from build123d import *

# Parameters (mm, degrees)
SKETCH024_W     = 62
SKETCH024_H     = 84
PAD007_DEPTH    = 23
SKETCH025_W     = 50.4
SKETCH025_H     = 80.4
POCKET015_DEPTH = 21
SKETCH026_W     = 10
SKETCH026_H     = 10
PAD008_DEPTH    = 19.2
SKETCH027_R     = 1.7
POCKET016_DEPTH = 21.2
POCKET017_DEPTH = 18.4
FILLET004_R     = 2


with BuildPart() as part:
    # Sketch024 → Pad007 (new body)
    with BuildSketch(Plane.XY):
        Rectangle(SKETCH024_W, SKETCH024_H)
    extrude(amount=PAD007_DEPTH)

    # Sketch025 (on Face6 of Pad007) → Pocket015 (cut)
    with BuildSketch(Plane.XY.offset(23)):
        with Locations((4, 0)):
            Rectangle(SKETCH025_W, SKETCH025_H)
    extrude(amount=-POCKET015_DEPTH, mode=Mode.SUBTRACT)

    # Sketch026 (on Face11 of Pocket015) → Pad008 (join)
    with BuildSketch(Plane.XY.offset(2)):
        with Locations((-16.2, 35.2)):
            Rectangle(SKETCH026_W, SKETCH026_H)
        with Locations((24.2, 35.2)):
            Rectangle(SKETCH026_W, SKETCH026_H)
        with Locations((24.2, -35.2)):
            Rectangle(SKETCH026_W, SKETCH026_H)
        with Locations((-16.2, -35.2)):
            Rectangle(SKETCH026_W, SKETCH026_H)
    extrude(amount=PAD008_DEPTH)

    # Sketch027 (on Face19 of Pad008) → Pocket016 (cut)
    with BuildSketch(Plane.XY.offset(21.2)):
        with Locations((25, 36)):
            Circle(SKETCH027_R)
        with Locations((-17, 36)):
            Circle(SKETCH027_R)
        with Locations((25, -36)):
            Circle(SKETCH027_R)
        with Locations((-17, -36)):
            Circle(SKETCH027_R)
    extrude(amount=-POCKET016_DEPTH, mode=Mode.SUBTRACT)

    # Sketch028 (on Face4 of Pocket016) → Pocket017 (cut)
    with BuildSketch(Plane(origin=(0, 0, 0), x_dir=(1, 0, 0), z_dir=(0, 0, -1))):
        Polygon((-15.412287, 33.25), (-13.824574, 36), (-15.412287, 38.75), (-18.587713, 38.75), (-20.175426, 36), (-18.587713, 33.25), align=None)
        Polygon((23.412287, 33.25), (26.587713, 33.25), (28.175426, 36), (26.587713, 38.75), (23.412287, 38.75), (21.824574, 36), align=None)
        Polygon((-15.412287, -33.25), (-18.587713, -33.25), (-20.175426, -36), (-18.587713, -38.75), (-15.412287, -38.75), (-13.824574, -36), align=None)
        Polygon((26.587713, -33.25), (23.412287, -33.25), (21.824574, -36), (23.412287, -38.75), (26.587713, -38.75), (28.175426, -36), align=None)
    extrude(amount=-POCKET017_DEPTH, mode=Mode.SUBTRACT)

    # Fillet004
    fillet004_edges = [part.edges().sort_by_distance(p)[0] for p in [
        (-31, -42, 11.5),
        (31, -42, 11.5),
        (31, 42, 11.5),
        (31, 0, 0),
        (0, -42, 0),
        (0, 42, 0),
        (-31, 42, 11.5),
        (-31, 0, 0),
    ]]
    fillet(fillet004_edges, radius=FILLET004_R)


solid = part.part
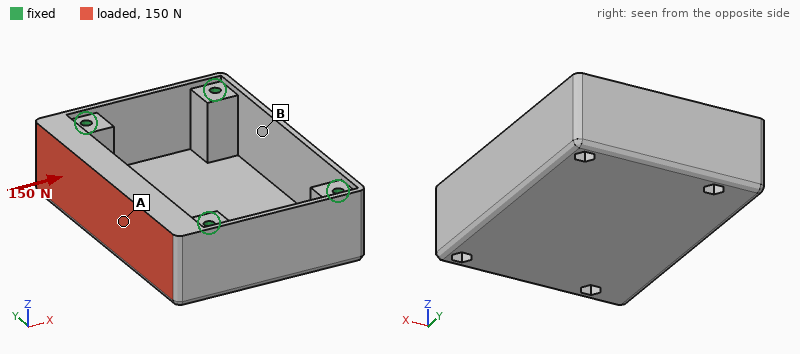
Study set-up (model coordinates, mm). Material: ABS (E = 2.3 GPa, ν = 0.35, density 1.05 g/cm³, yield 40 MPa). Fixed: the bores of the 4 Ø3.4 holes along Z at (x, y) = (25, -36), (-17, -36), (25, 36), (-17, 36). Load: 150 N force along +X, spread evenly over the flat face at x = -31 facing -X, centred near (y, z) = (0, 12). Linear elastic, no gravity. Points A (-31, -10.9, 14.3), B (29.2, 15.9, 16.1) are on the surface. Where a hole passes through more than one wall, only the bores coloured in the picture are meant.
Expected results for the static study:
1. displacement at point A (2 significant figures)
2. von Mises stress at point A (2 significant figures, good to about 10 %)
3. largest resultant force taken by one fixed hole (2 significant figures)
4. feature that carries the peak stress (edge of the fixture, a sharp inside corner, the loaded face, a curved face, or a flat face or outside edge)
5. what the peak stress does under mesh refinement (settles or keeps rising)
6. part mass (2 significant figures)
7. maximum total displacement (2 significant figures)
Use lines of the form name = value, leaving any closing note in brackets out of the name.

displacement at point A = 29 µm
von Mises stress at point A = 0.77 MPa
largest resultant force taken by one fixed hole = 67 N
feature that carries the peak stress = edge of the fixture
what the peak stress does under mesh refinement = keeps rising
part mass = 42 g
maximum total displacement = 39 µm
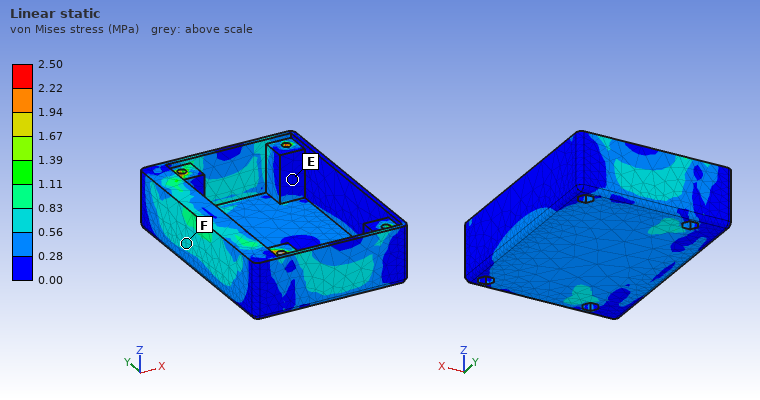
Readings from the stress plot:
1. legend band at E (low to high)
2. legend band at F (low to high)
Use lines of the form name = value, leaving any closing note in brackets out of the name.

legend band at E = 0.00 to 0.28 MPa
legend band at F = 0.56 to 0.83 MPa
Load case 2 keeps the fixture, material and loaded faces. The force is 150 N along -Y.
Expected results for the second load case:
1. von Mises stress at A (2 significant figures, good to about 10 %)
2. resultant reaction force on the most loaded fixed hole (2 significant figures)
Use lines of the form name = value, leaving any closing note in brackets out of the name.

von Mises stress at A = 0.46 MPa
resultant reaction force on the most loaded fixed hole = 73 N
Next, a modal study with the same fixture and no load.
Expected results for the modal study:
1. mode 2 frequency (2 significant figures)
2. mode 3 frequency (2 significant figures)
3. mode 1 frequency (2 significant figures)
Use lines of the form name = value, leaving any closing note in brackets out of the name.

mode 2 frequency = 1400 Hz
mode 3 frequency = 1900 Hz
mode 1 frequency = 1100 Hz
